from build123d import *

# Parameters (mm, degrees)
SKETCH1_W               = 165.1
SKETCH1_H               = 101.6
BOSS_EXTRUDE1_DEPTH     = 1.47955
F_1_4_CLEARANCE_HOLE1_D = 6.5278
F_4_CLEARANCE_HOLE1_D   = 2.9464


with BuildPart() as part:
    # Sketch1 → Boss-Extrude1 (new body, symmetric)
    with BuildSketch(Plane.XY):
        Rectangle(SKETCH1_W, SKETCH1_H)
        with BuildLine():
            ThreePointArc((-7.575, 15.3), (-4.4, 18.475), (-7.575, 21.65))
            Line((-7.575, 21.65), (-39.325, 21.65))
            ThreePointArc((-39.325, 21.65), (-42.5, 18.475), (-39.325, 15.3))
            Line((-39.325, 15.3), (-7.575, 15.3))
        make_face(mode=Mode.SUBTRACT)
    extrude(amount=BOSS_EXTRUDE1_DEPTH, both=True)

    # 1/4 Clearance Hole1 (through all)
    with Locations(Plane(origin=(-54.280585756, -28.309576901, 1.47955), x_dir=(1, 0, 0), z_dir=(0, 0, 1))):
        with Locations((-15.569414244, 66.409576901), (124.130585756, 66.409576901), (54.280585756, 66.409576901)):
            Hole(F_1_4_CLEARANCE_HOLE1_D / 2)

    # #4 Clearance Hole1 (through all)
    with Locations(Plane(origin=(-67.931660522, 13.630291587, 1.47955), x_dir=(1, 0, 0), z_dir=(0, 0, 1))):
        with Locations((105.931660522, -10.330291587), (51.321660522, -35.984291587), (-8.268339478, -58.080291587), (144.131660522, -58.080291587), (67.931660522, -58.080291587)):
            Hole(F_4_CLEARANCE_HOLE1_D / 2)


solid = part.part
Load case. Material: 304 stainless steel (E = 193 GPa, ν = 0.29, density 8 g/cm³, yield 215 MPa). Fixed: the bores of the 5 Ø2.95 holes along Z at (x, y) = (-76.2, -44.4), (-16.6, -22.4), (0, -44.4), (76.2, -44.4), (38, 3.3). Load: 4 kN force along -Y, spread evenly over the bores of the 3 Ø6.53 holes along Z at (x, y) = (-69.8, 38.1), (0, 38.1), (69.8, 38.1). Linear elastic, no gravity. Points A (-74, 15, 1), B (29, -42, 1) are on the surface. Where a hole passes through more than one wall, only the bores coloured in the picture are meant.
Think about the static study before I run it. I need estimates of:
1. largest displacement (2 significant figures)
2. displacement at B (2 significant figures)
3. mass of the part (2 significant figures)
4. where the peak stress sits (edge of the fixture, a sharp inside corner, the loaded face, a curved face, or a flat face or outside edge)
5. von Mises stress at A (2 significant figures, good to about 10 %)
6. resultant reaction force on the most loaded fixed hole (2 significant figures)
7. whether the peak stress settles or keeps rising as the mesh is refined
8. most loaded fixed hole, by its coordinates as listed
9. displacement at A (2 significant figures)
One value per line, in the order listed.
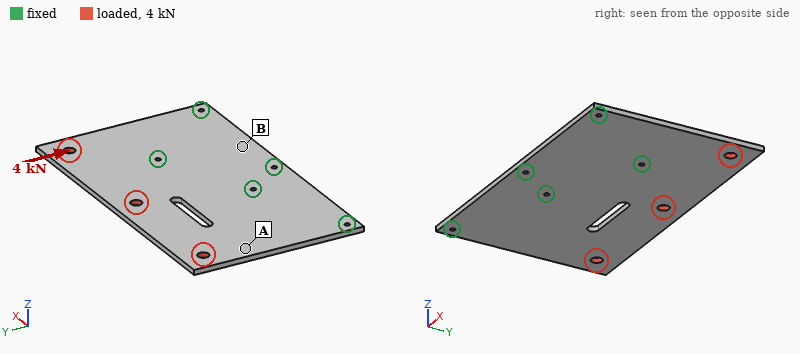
7.9 µm
1.2 µm
390 g
edge of the fixture
14 MPa
1.2 kN
keeps rising
(38, 3.3)
5.2 µm
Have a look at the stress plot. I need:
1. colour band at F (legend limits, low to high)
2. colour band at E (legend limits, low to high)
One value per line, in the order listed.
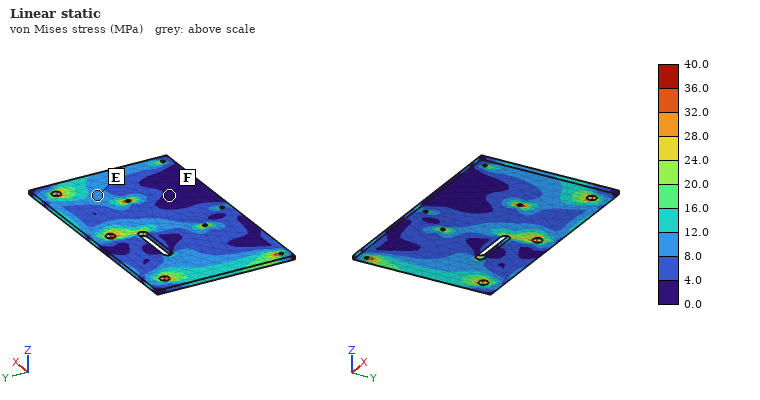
0.0 to 4.0 MPa
8.0 to 12.0 MPa
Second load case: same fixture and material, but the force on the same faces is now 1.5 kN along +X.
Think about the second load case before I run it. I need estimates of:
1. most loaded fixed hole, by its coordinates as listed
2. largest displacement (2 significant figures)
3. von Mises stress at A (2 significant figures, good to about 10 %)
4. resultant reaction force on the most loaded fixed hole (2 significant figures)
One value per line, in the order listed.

(38, 3.3)
6.2 µm
3.8 MPa
960 N
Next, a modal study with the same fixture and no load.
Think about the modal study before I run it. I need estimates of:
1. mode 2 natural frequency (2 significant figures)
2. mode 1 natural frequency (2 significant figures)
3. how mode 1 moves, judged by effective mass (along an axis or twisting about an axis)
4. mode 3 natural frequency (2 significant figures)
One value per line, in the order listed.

810 Hz
410 Hz
along Z
1000 Hz
